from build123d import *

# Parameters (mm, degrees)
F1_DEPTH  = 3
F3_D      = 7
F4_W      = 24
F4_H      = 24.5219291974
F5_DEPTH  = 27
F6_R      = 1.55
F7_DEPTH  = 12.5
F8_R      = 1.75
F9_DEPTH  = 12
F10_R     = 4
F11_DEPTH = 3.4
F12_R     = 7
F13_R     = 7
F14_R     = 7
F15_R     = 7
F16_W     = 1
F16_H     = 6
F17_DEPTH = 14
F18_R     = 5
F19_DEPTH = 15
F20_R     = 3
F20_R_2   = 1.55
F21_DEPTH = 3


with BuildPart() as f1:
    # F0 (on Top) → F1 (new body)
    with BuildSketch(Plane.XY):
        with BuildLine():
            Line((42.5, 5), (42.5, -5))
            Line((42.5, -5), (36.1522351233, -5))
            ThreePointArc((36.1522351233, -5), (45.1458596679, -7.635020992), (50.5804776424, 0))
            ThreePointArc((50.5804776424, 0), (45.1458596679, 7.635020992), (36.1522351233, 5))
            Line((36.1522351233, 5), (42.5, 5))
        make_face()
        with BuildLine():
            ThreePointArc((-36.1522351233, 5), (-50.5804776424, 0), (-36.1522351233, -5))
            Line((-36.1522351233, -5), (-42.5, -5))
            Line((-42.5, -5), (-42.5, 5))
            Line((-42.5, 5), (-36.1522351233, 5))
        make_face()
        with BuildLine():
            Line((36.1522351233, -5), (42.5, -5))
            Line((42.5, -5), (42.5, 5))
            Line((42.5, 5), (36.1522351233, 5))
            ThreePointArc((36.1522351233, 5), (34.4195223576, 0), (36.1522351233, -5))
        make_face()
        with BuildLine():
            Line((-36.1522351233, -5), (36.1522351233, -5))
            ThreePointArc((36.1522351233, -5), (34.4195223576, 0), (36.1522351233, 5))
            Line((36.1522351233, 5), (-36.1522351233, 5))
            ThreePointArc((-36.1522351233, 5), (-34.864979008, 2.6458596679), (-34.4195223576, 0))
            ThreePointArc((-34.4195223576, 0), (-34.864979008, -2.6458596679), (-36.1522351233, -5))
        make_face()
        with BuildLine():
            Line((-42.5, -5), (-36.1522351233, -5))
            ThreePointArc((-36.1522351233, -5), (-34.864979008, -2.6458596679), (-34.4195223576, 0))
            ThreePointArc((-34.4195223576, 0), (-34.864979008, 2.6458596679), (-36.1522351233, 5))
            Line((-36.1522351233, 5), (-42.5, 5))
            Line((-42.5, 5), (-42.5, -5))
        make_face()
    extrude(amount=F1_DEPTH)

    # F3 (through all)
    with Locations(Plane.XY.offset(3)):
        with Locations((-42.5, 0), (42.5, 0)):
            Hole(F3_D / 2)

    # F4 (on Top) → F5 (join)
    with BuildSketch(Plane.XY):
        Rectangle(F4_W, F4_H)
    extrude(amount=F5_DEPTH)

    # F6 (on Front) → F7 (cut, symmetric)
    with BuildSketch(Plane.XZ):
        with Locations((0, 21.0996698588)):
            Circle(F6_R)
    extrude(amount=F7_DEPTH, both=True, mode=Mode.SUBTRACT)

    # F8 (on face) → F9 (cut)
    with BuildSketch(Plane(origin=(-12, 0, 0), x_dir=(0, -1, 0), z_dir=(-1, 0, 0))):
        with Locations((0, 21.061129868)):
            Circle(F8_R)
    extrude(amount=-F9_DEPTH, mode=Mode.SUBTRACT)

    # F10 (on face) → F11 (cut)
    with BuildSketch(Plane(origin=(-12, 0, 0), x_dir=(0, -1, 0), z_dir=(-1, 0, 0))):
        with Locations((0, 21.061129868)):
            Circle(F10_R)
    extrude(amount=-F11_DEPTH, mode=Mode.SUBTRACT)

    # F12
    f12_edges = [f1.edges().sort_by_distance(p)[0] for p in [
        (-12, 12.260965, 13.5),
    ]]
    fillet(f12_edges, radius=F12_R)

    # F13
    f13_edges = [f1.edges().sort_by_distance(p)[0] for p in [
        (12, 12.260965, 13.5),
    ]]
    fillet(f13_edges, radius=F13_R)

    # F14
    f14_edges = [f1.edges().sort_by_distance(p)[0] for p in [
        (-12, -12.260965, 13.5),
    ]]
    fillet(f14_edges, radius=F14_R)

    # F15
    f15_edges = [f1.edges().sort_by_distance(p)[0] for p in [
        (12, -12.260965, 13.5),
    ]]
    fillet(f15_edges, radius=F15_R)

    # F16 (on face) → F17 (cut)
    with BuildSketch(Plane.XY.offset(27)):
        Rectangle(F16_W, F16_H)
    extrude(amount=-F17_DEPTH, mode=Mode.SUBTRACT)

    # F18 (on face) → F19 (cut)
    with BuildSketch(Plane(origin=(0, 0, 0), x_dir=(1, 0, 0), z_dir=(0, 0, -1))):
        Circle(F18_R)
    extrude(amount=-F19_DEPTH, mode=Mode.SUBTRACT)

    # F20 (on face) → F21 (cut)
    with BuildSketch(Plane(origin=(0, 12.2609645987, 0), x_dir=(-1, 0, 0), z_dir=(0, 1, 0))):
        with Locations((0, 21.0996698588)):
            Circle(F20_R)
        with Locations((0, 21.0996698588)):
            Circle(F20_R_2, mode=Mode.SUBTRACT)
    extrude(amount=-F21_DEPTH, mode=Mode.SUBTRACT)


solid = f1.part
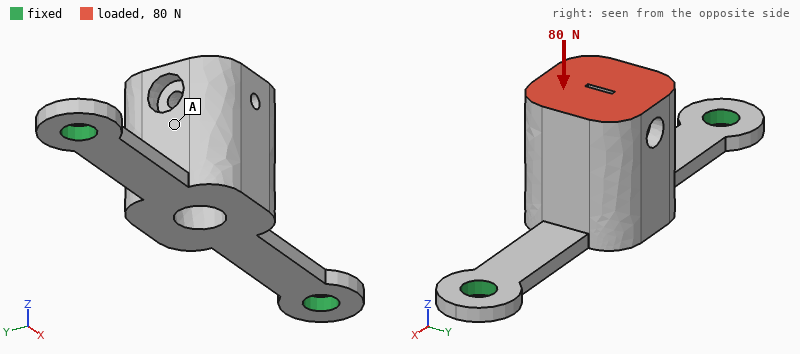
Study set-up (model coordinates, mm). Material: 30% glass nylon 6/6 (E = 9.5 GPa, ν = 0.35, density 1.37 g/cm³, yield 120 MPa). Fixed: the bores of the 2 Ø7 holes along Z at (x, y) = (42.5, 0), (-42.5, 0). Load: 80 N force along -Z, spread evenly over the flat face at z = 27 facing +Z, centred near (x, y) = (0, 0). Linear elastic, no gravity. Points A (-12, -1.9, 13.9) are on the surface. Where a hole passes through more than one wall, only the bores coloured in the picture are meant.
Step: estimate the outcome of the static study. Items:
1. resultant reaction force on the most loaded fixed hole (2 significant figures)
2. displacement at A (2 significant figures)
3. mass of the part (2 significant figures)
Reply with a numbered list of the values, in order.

1. 47 N
2. 0.36 mm
3. 21 g
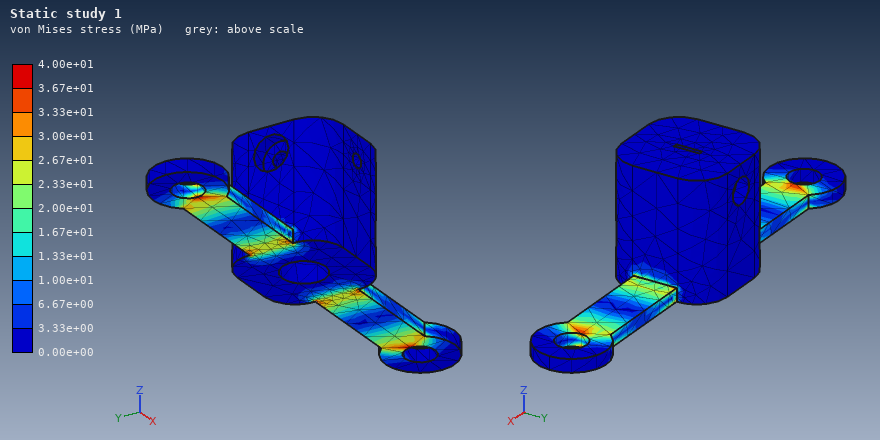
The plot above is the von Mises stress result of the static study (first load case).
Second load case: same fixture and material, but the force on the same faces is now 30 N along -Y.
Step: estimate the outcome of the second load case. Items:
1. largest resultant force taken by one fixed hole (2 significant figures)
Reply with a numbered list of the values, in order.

1. 15 N
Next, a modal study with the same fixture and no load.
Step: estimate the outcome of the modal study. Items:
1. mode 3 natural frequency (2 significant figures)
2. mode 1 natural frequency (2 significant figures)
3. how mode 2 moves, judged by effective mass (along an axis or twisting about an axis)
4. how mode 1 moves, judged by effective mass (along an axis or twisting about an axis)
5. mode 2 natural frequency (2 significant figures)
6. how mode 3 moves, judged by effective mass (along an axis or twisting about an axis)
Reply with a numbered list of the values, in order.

1. 890 Hz
2. 330 Hz
3. along Z
4. along Y
5. 550 Hz
6. along X
